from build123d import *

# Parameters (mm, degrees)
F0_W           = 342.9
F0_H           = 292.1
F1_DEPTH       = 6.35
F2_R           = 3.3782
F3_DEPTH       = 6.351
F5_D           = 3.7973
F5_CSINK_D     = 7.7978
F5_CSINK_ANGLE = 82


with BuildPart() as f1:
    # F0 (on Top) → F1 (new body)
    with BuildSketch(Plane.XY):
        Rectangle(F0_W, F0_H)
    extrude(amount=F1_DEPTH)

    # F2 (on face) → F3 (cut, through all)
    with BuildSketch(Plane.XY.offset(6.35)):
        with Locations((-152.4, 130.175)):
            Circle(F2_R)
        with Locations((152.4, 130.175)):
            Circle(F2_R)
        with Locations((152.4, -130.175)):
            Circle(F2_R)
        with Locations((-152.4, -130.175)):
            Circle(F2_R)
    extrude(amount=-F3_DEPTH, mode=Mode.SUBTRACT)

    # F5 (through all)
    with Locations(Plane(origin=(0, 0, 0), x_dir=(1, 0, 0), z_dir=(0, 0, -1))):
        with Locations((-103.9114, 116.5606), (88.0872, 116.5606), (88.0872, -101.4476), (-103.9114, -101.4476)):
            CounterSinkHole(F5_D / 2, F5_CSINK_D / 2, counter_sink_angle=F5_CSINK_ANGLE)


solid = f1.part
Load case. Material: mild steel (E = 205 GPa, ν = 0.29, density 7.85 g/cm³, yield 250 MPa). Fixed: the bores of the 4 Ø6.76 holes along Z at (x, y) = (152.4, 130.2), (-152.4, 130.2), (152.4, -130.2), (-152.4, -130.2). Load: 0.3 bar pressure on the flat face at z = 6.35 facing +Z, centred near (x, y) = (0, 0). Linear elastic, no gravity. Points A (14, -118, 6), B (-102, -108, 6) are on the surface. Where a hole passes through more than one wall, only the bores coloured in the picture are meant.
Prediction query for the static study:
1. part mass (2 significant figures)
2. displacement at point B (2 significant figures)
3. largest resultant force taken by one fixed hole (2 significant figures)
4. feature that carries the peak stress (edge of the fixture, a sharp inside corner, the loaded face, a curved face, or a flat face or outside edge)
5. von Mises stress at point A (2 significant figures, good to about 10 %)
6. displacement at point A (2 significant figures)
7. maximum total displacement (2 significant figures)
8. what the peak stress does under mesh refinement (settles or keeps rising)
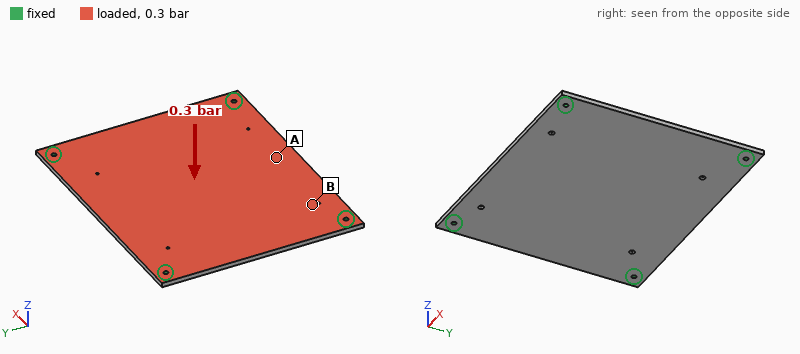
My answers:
5.0 kg
0.13 mm
750 N
edge of the fixture
25 MPa
0.28 mm
0.38 mm
keeps rising
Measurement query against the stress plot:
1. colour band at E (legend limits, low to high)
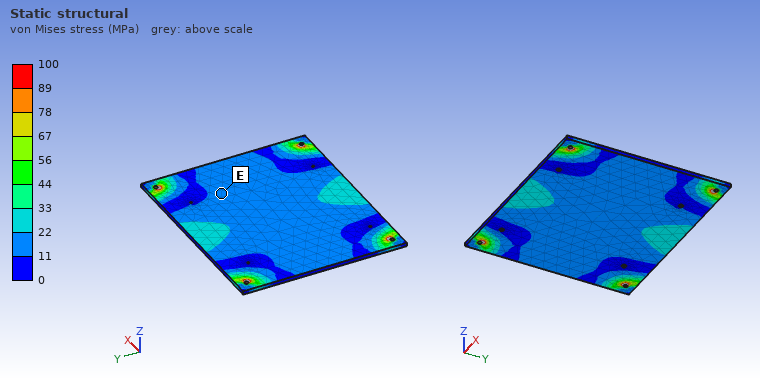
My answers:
11 to 22 MPa
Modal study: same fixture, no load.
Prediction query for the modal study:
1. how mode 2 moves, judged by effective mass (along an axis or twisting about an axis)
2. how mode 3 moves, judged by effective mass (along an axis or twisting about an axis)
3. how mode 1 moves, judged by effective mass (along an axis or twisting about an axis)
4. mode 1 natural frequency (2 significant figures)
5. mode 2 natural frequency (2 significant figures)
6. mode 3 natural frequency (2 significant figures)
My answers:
twisting about X
twisting about Y
along Z
240 Hz
410 Hz
480 Hz
